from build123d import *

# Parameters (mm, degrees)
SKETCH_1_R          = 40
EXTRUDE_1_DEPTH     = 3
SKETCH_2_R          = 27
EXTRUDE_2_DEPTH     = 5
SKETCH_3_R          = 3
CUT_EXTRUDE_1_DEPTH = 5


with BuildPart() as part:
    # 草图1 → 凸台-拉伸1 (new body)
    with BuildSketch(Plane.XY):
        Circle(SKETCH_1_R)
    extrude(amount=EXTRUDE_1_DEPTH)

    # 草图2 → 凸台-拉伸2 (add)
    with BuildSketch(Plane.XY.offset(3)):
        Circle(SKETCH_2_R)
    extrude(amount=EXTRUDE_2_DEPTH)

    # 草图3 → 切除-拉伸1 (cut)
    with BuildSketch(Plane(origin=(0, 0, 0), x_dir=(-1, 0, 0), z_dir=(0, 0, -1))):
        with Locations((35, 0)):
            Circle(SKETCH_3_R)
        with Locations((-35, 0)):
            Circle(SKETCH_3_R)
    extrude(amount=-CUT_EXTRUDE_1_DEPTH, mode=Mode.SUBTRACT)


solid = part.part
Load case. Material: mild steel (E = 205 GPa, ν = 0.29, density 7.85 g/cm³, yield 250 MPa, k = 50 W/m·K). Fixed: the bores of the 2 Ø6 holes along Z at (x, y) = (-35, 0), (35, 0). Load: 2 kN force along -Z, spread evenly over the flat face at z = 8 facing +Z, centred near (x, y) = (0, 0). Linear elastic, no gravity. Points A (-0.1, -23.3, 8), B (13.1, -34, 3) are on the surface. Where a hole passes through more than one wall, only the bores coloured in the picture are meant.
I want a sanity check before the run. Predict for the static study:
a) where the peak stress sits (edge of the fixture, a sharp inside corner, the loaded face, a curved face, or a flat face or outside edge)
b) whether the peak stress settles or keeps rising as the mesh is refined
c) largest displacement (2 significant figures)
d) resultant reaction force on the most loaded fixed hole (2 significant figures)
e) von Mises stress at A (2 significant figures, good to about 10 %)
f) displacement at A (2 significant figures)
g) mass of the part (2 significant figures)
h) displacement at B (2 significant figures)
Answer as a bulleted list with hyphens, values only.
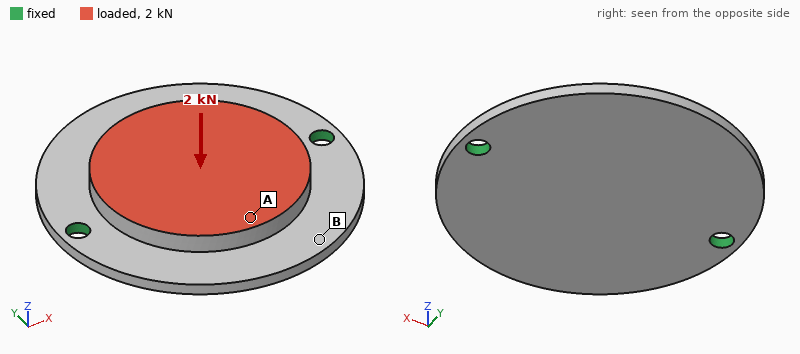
- edge of the fixture
- keeps rising
- 30 µm
- 1.7 kN
- 22 MPa
- 24 µm
- 210 g
- 26 µm
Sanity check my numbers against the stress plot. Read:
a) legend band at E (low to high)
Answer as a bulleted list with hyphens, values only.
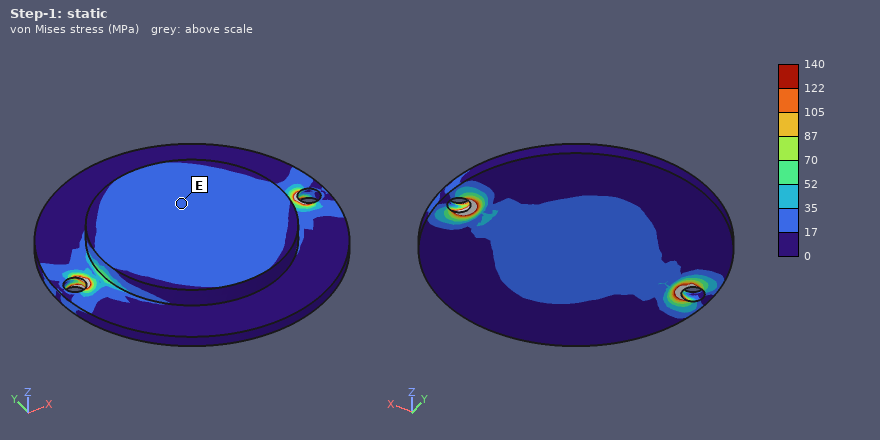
- 17 to 35 MPa
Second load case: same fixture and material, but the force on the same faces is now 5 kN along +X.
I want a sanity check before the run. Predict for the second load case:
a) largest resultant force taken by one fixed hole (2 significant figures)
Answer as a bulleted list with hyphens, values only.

- 2.6 kN
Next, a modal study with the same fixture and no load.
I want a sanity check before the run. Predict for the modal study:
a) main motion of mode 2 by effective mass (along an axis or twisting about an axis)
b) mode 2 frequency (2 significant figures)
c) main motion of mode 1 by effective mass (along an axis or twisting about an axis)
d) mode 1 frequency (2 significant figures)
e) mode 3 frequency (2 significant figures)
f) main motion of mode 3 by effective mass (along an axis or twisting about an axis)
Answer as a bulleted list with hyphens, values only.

- along Z
- 3500 Hz
- twisting about X
- 1600 Hz
- 7400 Hz
- twisting about Y
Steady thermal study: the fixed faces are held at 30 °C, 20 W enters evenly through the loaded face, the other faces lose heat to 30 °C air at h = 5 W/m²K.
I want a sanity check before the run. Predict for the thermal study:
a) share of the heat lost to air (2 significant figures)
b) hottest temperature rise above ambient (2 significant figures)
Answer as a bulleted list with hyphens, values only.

- 5.9 %
- 32 K
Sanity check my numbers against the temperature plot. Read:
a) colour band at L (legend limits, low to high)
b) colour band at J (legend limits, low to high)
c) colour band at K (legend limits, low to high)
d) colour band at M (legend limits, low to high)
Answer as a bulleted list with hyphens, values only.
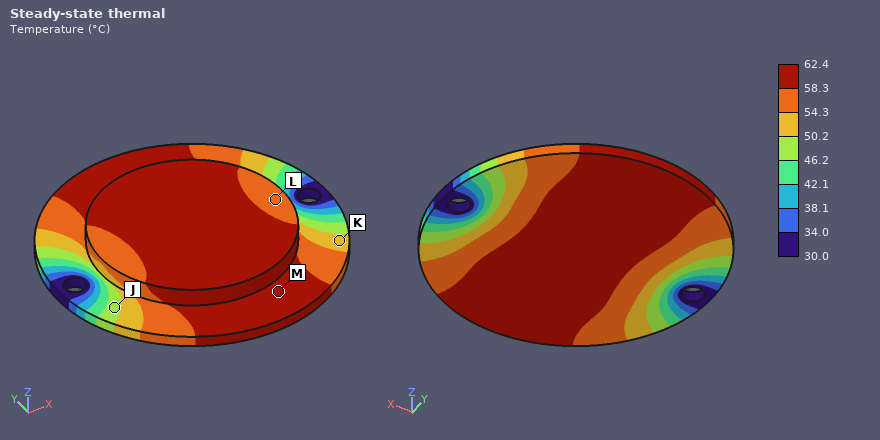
- 54.3 to 58.3 °C
- 46.2 to 50.2 °C
- 50.2 to 54.3 °C
- 58.3 to 62.4 °C
